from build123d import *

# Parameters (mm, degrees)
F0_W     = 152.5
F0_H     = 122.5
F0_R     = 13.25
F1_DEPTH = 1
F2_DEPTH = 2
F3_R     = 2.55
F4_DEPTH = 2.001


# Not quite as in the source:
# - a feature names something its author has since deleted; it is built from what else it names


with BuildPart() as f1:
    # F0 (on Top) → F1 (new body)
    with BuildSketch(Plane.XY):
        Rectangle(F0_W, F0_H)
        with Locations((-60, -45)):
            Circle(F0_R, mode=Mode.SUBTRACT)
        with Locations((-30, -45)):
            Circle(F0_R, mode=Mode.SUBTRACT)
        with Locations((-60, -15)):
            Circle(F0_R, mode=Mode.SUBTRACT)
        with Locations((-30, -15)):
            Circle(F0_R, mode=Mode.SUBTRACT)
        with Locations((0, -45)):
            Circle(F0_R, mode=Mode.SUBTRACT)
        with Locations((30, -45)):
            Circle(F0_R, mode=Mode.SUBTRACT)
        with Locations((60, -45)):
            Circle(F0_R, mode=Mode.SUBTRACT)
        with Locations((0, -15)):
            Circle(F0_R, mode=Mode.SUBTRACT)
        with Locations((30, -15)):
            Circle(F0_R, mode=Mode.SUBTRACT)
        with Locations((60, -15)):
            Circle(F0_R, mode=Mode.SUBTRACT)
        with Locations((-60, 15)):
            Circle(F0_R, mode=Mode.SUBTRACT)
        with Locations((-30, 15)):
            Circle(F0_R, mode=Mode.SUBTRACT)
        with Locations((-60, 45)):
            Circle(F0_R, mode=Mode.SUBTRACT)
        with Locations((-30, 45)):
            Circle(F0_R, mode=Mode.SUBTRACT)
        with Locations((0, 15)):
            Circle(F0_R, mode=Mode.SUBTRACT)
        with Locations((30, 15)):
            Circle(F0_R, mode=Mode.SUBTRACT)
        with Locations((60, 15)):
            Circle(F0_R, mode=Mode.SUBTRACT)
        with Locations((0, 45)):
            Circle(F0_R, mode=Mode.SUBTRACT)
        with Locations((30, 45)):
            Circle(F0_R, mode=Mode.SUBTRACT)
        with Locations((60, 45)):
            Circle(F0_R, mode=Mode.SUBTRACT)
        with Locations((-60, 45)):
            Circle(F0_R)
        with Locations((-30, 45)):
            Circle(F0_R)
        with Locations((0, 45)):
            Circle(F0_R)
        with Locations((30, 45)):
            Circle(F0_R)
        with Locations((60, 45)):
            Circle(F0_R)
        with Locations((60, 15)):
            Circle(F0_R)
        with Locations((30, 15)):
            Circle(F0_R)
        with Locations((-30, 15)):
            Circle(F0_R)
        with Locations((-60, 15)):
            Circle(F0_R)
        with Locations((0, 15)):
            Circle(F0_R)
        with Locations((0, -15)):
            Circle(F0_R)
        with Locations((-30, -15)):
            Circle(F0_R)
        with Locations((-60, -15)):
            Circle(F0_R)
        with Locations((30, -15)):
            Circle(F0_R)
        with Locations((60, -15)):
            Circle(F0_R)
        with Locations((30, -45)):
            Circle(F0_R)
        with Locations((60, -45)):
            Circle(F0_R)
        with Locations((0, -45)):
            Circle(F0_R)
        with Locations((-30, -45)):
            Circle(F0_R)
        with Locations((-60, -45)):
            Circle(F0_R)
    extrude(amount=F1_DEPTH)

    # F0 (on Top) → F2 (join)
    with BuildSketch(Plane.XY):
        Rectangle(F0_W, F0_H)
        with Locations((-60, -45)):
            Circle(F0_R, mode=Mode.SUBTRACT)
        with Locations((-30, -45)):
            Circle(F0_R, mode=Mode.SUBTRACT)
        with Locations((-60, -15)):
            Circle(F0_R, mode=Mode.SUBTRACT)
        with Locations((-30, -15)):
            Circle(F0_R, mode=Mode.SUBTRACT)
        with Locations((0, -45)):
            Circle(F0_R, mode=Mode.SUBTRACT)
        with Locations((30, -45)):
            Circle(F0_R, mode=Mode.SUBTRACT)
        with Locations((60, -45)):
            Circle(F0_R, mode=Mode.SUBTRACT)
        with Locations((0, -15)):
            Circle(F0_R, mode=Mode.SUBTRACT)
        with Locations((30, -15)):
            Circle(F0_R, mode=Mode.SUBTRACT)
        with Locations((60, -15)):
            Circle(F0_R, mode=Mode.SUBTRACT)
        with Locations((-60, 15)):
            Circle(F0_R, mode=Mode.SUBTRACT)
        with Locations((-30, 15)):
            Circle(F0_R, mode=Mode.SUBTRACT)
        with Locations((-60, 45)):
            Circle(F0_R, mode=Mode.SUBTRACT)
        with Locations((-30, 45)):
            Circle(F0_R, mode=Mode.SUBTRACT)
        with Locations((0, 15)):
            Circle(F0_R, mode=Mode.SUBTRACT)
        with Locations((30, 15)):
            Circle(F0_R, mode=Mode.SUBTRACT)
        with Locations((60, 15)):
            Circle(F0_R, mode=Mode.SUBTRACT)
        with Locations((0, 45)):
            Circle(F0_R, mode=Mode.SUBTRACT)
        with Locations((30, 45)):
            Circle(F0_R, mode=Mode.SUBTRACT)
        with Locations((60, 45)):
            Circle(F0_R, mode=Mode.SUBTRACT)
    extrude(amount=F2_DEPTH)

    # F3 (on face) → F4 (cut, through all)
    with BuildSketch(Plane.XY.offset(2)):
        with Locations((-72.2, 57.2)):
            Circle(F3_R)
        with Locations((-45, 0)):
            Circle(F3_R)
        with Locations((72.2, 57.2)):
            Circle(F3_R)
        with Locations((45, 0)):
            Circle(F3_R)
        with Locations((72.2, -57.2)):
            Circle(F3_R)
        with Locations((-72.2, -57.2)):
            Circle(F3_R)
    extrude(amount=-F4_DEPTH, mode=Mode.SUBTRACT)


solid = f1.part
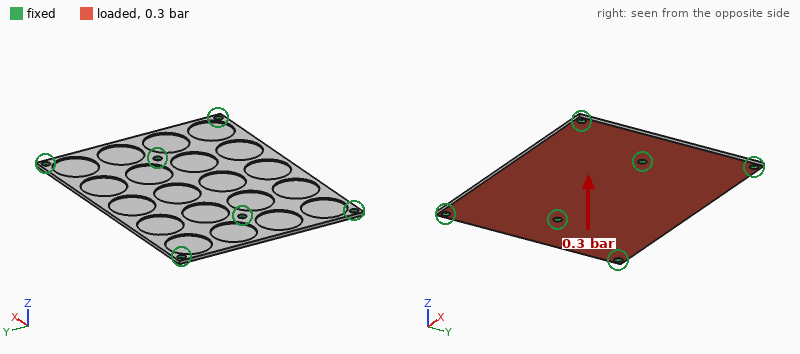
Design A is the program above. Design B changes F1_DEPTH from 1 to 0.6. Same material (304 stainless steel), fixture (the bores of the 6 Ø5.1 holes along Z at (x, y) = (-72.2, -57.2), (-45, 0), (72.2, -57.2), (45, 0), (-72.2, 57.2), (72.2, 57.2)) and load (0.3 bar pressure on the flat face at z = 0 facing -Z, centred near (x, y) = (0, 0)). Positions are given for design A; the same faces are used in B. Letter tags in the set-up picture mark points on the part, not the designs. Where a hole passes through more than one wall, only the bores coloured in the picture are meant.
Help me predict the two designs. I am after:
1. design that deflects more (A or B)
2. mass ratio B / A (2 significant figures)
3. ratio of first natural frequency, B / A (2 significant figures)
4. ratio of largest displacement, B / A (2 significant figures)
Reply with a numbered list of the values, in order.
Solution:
1. B
2. 0.83
3. 1.0
4. 1.1
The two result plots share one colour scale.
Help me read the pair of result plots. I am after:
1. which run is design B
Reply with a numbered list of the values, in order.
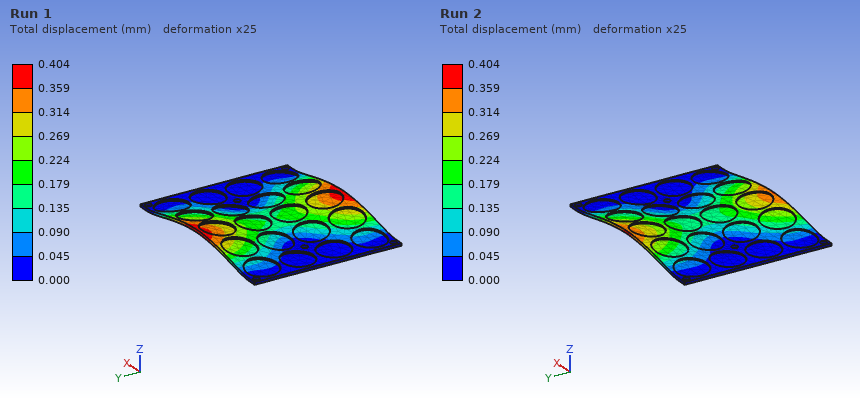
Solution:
1. Run 1
